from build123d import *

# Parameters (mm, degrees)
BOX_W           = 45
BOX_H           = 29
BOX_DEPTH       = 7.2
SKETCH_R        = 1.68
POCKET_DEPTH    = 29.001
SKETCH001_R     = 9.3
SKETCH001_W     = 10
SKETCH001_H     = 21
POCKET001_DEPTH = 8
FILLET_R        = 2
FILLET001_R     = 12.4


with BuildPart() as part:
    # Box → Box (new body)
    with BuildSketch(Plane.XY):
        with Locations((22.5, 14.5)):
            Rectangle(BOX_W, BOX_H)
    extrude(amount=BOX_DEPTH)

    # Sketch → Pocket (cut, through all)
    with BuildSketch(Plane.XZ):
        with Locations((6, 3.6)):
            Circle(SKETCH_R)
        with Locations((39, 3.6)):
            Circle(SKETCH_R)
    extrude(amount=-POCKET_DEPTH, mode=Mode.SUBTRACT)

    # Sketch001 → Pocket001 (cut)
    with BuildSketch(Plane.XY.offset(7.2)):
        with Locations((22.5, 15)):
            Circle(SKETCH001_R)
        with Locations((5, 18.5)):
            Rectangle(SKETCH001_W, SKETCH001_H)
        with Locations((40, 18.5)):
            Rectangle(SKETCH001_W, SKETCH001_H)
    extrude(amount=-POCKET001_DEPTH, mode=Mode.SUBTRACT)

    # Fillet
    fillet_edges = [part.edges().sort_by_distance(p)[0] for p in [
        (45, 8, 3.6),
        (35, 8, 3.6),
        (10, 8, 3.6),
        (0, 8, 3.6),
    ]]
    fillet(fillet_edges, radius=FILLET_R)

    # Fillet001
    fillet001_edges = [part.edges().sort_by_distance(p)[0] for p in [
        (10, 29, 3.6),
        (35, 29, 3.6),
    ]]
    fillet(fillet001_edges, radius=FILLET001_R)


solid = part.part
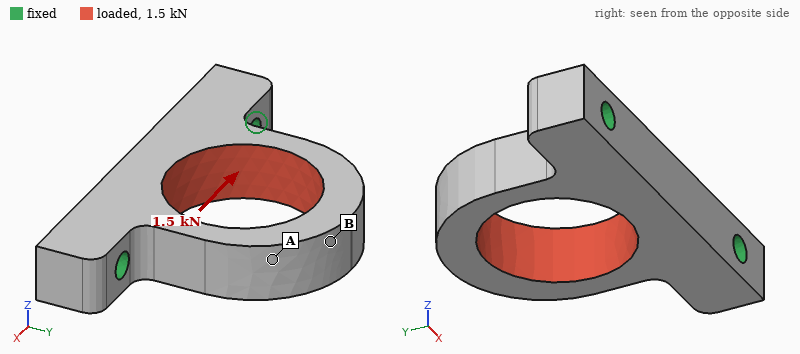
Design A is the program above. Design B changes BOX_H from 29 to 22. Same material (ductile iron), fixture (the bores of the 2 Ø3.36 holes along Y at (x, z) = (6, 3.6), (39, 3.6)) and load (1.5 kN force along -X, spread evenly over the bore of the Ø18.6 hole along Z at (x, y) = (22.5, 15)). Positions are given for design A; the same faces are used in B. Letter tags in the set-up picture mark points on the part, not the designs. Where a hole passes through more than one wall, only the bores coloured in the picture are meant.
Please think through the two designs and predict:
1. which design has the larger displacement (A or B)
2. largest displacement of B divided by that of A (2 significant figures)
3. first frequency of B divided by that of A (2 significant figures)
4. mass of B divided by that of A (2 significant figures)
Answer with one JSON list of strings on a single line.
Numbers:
["B", "2.5", "1.5", "0.55"]
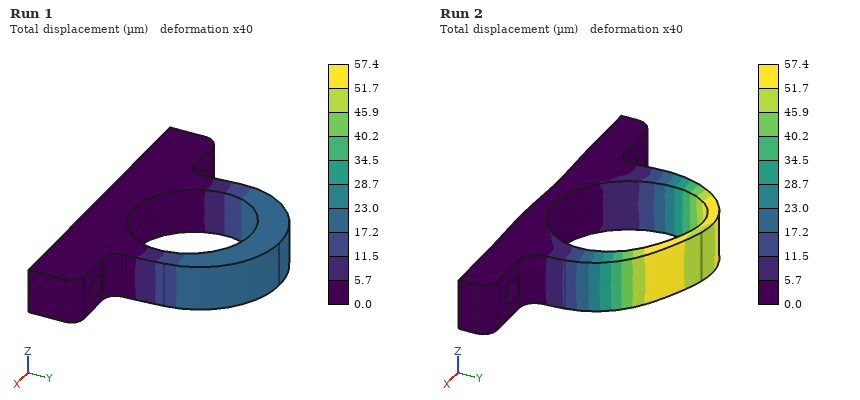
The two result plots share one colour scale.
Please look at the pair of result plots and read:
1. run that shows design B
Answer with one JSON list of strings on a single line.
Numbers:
["Run 2"]
